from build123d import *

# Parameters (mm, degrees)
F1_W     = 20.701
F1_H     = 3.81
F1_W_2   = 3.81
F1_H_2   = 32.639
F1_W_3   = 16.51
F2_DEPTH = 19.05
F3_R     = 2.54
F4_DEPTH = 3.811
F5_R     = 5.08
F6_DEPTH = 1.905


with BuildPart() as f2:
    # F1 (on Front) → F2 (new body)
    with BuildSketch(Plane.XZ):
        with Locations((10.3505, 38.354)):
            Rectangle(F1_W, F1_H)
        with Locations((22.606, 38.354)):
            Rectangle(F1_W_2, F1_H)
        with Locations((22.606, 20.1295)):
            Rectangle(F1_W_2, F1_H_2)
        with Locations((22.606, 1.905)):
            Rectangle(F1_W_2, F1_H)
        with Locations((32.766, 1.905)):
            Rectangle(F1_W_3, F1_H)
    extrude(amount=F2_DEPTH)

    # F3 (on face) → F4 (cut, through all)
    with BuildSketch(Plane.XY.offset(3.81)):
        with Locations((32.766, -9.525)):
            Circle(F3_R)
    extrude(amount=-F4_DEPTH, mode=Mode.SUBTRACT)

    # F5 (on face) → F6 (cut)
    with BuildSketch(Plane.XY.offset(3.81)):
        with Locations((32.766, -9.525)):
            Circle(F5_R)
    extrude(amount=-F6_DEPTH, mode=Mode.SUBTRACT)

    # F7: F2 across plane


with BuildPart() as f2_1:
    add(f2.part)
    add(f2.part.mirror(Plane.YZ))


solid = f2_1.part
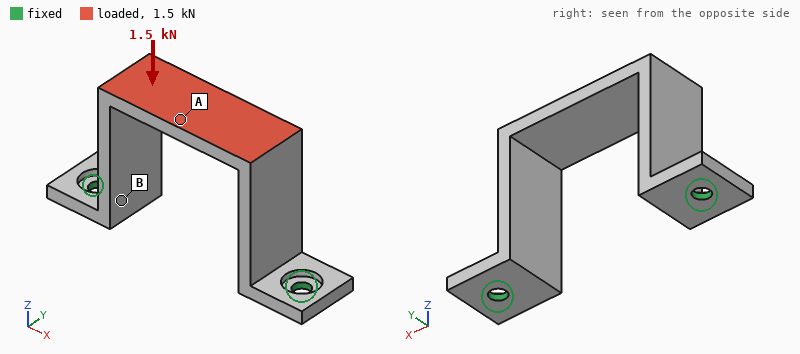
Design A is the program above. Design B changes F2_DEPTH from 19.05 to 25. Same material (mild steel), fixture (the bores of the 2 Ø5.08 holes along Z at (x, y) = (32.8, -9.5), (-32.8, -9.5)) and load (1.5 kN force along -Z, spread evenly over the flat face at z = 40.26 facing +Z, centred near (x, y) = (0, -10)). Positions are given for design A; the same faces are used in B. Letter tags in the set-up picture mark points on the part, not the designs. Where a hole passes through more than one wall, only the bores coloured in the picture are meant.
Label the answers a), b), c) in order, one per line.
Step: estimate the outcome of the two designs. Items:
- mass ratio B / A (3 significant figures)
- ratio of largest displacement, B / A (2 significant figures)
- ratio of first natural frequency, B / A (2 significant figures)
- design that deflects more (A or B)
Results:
a) 1.32
b) 1.4
c) 0.91
d) B
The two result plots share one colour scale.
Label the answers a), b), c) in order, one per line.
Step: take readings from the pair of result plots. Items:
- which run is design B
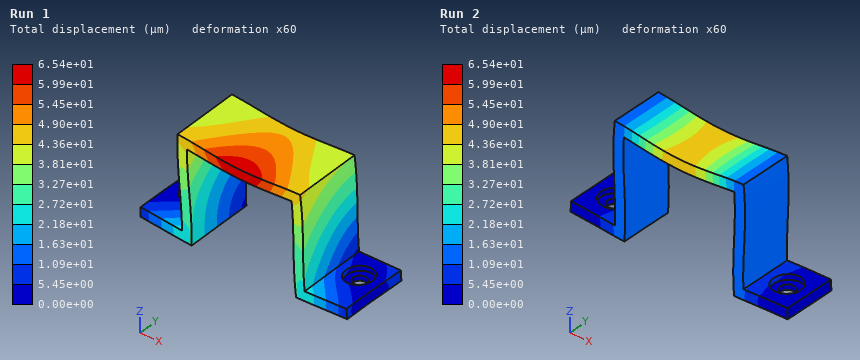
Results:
a) Run 1
